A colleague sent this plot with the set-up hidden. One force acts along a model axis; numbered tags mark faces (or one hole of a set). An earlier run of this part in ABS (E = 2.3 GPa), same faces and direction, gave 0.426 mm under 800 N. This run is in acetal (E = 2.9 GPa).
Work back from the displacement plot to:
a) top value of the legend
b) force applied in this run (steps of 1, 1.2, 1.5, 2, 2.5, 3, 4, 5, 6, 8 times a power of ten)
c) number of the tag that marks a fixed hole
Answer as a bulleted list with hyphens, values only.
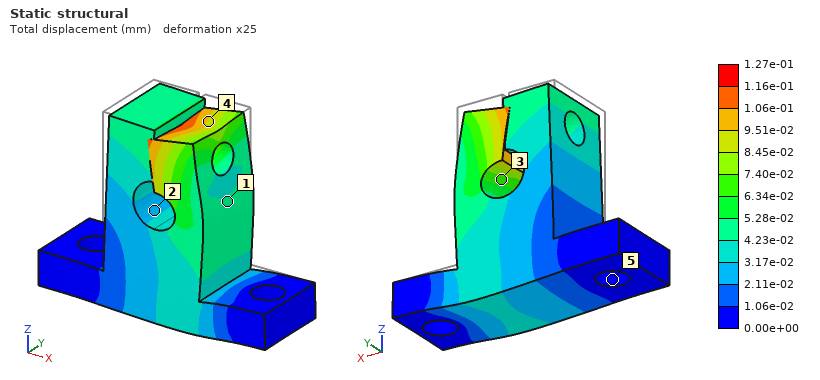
- 1.27e-01 mm
- 300 N
- 5
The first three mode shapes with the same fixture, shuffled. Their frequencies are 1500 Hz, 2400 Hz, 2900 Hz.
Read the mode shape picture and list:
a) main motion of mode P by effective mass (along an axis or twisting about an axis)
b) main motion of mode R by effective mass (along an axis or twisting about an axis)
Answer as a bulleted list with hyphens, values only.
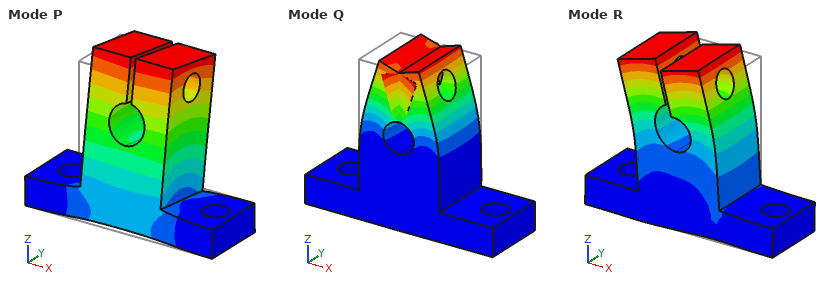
- along Y
- along X
